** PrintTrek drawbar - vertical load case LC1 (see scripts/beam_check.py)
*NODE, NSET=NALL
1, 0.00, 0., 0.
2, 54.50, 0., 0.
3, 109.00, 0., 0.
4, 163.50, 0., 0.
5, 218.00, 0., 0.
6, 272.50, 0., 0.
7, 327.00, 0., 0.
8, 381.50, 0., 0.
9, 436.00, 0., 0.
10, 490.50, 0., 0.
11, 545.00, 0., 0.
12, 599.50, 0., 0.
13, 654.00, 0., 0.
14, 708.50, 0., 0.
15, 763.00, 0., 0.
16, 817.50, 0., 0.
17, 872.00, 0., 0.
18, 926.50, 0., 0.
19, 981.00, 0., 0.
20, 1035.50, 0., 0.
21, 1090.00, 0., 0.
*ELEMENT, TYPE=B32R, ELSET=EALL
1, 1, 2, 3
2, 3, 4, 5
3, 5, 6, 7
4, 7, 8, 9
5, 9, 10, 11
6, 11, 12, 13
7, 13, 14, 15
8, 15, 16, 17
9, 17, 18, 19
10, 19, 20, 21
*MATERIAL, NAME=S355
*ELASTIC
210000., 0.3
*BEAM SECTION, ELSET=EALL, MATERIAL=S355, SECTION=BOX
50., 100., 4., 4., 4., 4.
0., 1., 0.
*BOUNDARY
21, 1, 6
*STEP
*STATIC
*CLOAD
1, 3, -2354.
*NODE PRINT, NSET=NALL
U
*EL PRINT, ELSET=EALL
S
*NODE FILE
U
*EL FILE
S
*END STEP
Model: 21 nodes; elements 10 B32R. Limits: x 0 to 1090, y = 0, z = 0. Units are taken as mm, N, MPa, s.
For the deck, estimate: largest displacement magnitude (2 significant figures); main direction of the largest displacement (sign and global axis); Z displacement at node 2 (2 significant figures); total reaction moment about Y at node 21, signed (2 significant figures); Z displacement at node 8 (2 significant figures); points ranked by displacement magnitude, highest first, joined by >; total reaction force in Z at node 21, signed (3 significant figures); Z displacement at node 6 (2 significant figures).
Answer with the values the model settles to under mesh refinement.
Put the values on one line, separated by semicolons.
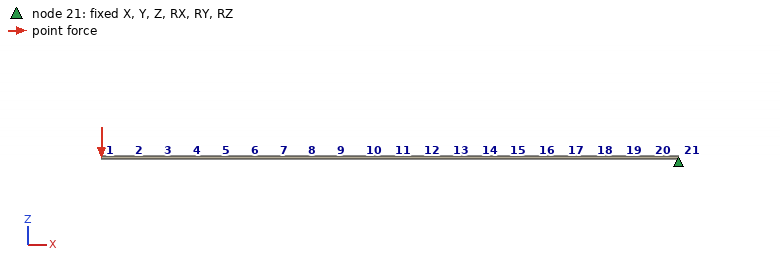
3.4 mm; -Z; -3.1 mm; 2.6e+06 N·mm; -1.7 mm; node 2 > node 6 > node 8 > node 12 > node 21; 2350 N; -2.2 mm
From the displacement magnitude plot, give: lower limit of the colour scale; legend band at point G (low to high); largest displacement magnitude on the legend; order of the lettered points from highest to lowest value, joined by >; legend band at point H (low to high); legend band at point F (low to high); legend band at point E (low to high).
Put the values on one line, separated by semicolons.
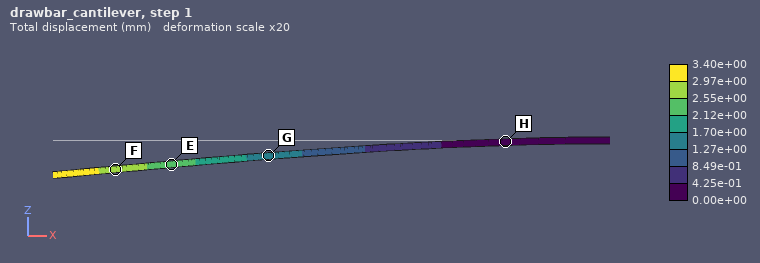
0.00e+00 mm; 1.27e+00 to 1.70e+00 mm; 3.40e+00 mm; F > E > G > H; 0.00e+00 to 4.25e-01 mm; 2.55e+00 to 2.97e+00 mm; 2.12e+00 to 2.55e+00 mm
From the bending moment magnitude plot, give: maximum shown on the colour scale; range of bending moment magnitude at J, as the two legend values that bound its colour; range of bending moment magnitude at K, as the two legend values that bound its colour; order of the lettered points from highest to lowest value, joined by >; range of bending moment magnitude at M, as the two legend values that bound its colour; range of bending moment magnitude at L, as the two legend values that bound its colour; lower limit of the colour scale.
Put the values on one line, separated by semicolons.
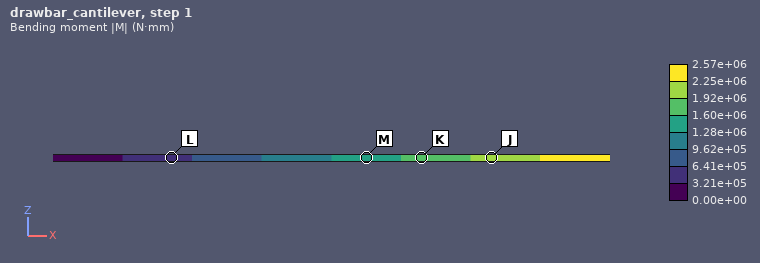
2.57e+06 N·mm; 1.92e+06 to 2.25e+06 N·mm; 1.60e+06 to 1.92e+06 N·mm; J > K > M > L; 1.28e+06 to 1.60e+06 N·mm; 3.21e+05 to 6.41e+05 N·mm; 0.00e+00 N·mm
